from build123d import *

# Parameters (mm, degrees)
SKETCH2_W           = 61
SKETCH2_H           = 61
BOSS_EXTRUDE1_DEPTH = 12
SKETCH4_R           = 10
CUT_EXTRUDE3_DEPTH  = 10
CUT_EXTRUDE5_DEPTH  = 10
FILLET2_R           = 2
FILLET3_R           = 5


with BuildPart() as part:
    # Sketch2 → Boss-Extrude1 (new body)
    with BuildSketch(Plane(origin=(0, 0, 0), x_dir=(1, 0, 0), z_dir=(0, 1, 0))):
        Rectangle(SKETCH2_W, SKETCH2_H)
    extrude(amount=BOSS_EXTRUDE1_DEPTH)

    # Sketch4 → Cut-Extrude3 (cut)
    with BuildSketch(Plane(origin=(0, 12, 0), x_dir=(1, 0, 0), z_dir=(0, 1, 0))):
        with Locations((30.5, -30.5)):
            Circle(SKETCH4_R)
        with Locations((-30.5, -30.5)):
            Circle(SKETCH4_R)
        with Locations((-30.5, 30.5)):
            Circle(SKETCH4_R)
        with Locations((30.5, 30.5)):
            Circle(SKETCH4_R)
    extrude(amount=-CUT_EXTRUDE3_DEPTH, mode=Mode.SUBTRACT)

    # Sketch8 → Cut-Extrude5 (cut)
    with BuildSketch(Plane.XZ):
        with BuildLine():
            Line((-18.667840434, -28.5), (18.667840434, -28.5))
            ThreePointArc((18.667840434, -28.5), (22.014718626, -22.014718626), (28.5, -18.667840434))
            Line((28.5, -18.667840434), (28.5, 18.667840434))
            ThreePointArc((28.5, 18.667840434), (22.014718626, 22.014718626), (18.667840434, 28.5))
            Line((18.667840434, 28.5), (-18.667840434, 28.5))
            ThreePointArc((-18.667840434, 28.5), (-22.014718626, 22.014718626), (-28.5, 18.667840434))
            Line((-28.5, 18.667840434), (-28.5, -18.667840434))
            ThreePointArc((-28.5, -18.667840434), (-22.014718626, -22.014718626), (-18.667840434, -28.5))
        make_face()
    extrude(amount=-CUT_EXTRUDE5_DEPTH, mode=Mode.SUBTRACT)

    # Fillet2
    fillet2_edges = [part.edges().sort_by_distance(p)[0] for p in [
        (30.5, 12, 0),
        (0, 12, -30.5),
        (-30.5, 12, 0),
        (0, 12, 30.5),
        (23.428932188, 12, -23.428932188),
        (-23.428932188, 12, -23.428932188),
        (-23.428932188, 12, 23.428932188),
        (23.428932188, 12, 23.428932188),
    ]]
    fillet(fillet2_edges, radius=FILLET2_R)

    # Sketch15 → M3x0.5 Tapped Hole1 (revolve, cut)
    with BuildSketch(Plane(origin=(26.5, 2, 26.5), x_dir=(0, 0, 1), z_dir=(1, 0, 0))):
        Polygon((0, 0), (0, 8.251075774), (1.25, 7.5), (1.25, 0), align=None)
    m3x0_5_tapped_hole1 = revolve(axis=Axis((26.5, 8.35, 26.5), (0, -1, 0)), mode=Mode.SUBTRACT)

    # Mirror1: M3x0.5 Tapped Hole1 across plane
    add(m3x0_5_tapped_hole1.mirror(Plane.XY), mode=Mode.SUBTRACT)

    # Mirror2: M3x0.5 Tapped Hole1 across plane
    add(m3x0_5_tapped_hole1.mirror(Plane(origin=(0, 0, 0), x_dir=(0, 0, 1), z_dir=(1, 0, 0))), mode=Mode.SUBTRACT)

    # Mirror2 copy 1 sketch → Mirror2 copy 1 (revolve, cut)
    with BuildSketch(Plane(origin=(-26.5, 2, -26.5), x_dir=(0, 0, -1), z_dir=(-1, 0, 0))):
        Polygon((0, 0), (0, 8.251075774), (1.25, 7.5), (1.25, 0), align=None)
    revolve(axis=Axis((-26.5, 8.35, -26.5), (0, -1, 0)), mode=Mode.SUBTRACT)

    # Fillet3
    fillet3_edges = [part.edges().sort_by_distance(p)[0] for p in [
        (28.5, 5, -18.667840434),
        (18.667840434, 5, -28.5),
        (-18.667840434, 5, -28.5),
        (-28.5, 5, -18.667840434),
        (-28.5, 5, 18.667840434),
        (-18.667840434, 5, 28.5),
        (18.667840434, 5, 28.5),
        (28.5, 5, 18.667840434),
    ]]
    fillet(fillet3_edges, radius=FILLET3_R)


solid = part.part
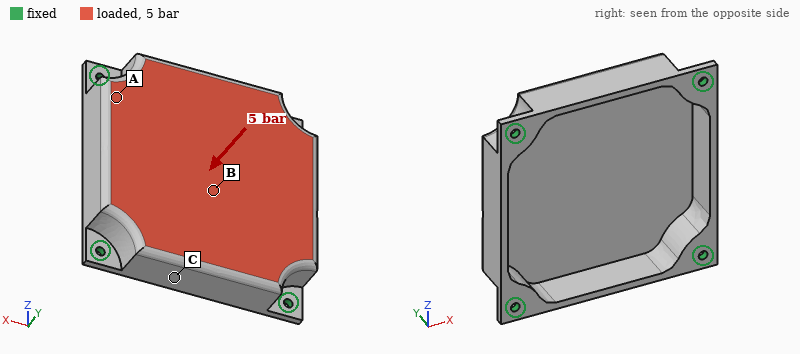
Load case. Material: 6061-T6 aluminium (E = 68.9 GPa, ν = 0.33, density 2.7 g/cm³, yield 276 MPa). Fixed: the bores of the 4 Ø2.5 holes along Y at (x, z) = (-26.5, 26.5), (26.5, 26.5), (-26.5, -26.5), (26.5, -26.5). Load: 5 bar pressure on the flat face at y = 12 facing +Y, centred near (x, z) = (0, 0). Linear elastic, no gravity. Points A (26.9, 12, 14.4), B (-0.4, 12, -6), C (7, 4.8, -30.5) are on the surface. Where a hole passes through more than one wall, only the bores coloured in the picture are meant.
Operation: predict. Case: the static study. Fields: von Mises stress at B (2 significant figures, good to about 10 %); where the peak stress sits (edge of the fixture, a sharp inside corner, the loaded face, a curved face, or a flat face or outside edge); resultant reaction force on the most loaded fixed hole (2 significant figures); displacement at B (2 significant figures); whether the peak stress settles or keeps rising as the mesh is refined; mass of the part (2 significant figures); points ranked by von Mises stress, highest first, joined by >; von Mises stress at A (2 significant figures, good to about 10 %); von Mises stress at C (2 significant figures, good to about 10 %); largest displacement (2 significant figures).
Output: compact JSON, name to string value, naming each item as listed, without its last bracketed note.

{"von Mises stress at B": "74 MPa", "where the peak stress sits": "edge of the fixture", "resultant reaction force on the most loaded fixed hole": "470 N", "displacement at B": "0.21 mm", "whether the peak stress settles or keeps rising as the mesh is refined": "keeps rising", "mass of the part": "32 g", "points ranked by von Mises stress, highest first, joined by >": "B > A > C", "von Mises stress at A": "57 MPa", "von Mises stress at C": "28 MPa", "largest displacement": "0.23 mm"}
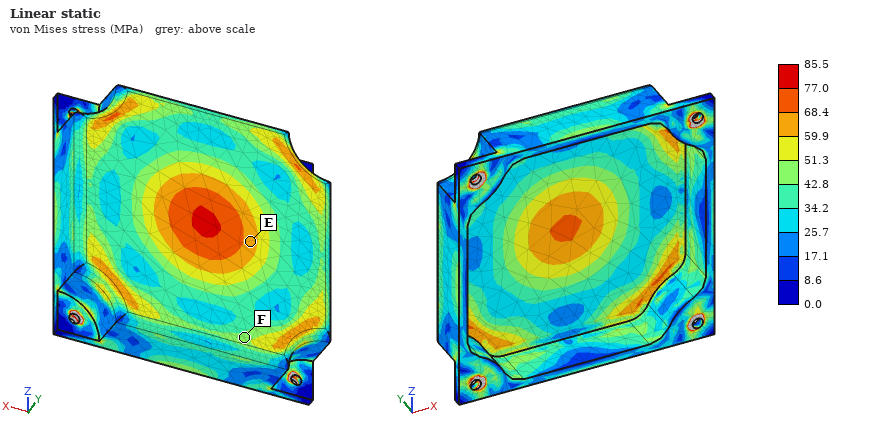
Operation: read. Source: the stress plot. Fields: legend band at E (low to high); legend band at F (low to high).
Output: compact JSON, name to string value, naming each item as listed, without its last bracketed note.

{"legend band at E": "59.9 to 68.4 MPa", "legend band at F": "42.8 to 51.3 MPa"}
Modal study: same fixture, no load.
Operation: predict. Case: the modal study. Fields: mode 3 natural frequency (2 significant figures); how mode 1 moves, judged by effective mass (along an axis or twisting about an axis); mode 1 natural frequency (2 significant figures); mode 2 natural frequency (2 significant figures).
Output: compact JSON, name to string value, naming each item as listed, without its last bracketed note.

{"mode 3 natural frequency": "7900 Hz", "how mode 1 moves, judged by effective mass": "along Y", "mode 1 natural frequency": "4000 Hz", "mode 2 natural frequency": "7900 Hz"}
